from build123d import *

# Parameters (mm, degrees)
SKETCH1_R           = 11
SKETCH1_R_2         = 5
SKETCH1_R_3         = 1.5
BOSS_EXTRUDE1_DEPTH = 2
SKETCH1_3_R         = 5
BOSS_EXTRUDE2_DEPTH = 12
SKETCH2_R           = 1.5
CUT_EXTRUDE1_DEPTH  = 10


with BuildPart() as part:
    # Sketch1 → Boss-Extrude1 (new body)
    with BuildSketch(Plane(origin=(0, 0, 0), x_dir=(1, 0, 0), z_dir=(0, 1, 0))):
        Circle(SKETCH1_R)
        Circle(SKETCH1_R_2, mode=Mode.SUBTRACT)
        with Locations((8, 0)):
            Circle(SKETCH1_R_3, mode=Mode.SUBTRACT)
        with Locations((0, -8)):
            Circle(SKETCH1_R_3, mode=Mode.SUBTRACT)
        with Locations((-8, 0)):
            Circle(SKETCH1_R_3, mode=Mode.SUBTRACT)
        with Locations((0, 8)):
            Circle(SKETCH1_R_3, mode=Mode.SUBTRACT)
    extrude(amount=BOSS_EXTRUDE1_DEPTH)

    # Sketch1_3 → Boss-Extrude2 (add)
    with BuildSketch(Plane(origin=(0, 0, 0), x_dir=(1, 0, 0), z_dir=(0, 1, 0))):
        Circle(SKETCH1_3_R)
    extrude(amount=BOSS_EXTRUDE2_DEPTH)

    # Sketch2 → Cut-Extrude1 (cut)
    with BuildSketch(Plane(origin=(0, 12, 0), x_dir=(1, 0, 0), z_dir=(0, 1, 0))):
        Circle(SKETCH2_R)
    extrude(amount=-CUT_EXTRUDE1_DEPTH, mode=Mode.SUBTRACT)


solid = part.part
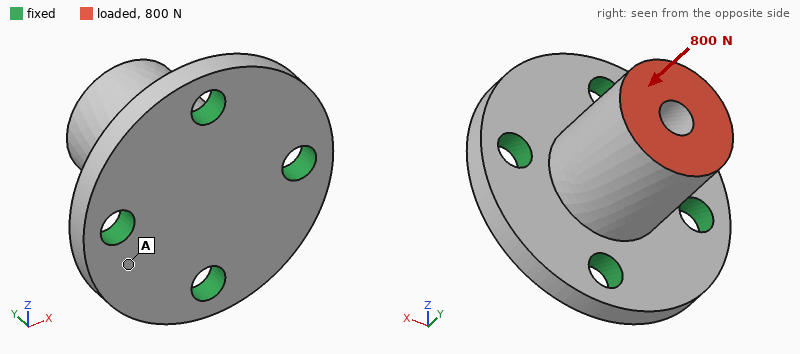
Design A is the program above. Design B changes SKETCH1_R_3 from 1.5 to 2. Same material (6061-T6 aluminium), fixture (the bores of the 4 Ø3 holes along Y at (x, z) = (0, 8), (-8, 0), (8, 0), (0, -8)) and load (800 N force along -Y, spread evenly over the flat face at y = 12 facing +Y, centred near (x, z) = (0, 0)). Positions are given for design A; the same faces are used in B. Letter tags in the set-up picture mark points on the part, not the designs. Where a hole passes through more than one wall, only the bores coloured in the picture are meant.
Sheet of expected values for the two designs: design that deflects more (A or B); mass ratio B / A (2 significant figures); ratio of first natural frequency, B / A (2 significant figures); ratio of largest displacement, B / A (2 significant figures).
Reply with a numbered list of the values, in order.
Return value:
1. A
2. 0.97
3. 1.1
4. 0.79
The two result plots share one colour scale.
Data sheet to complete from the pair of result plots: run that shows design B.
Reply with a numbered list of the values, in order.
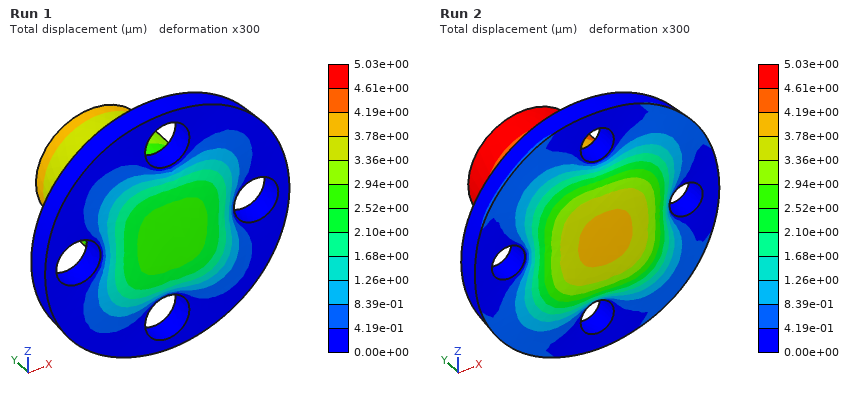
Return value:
1. Run 1
